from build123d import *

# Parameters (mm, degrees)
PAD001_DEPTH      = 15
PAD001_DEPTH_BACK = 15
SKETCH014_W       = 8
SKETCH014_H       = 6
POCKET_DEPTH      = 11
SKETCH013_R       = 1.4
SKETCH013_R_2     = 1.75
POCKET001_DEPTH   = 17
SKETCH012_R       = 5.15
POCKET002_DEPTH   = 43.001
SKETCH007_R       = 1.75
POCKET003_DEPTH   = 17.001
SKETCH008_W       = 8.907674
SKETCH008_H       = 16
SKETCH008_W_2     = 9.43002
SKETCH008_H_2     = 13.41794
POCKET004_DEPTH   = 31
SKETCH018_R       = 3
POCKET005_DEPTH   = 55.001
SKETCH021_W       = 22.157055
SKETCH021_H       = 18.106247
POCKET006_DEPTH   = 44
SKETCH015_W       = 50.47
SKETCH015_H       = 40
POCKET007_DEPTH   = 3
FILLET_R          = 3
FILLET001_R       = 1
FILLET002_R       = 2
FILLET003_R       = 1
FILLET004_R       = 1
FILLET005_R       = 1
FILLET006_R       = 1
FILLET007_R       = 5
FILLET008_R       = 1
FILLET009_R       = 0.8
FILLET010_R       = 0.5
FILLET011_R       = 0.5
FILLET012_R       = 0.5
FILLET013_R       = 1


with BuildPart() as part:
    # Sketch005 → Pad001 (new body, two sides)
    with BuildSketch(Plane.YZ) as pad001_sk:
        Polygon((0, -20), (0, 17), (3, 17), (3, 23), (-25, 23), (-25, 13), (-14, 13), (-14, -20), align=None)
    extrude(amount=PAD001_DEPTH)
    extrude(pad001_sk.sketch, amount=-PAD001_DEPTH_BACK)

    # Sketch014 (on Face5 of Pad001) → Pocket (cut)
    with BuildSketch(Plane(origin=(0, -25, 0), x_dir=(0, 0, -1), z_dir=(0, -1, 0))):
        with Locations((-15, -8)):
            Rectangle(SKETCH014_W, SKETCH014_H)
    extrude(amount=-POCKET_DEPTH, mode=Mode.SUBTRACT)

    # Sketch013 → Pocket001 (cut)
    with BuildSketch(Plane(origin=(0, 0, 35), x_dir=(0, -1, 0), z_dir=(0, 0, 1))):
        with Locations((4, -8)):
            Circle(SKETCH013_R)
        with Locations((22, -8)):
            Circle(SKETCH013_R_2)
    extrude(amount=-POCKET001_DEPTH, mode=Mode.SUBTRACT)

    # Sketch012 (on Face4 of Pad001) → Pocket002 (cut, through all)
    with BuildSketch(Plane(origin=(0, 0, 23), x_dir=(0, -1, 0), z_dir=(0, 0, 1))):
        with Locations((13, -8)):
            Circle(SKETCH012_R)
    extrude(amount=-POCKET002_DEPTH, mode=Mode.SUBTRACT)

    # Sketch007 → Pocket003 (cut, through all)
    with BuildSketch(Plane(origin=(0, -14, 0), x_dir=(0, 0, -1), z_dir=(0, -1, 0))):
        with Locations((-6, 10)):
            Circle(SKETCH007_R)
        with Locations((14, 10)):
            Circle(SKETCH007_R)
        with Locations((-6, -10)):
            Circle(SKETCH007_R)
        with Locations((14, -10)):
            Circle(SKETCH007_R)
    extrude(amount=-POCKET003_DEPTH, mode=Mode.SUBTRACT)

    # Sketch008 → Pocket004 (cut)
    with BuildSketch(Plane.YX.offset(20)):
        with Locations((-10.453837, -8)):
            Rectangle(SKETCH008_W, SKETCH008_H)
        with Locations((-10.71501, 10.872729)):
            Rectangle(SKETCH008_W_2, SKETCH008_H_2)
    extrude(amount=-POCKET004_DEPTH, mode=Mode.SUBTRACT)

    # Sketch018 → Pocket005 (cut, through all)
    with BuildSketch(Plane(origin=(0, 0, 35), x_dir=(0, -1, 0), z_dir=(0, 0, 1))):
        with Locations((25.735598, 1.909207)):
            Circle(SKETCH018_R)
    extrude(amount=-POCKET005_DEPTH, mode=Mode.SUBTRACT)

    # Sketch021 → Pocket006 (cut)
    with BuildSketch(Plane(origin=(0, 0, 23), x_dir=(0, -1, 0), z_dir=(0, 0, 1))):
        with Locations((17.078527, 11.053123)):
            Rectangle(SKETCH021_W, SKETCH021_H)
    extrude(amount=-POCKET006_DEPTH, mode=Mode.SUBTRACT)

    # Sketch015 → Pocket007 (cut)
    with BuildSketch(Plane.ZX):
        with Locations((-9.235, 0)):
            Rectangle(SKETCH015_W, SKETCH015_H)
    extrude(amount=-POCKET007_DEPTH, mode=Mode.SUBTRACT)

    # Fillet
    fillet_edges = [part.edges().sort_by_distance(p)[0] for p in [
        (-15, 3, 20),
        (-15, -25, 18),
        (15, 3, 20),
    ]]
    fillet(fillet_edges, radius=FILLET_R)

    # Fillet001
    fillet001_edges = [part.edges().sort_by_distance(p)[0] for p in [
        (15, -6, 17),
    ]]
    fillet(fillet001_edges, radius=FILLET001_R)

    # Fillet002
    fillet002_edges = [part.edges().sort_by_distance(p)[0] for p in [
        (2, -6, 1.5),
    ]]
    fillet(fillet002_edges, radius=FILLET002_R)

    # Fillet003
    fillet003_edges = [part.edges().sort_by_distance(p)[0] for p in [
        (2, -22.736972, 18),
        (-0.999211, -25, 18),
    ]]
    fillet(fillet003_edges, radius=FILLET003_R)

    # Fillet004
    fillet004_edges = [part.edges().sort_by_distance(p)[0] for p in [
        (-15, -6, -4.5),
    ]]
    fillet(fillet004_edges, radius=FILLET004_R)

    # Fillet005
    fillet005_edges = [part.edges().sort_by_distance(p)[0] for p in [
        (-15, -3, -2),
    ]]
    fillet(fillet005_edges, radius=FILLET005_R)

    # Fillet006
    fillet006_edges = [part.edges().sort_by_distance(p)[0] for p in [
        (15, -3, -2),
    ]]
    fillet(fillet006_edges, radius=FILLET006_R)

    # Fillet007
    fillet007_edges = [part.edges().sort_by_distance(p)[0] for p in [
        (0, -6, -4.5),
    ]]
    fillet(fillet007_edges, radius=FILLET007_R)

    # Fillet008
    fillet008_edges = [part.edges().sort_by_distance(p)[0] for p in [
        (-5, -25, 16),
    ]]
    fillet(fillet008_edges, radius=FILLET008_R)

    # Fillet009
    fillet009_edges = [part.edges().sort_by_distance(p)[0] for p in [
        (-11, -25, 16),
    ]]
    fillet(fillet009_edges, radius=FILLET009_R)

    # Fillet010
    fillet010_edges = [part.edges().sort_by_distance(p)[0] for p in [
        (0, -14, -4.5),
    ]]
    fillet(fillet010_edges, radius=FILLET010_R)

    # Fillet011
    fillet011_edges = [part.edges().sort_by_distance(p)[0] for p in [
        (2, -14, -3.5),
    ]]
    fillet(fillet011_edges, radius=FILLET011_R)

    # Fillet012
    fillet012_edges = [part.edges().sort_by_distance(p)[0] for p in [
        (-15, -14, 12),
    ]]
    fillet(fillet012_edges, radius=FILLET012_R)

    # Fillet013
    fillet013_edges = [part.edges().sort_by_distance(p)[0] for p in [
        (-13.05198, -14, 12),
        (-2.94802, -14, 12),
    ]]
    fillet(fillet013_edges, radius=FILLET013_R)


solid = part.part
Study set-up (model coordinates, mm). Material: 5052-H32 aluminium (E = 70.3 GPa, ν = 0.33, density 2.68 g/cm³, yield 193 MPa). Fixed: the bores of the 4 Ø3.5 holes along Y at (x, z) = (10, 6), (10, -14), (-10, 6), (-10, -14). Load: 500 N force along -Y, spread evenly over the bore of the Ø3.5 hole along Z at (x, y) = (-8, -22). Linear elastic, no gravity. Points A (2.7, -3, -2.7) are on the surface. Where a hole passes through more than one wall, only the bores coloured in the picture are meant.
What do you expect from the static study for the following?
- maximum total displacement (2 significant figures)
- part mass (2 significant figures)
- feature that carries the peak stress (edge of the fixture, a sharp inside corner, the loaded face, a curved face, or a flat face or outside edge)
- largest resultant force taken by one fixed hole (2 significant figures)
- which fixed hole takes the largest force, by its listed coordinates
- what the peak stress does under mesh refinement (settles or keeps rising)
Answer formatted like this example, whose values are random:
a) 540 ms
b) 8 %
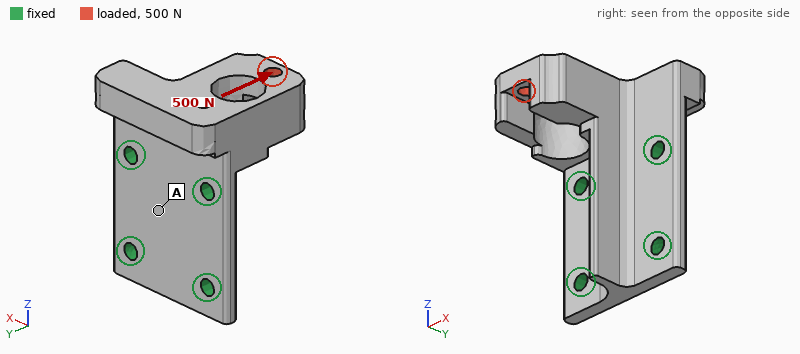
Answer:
a) 83 µm
b) 21 g
c) edge of the fixture
d) 580 N
e) (-10, 6)
f) keeps rising
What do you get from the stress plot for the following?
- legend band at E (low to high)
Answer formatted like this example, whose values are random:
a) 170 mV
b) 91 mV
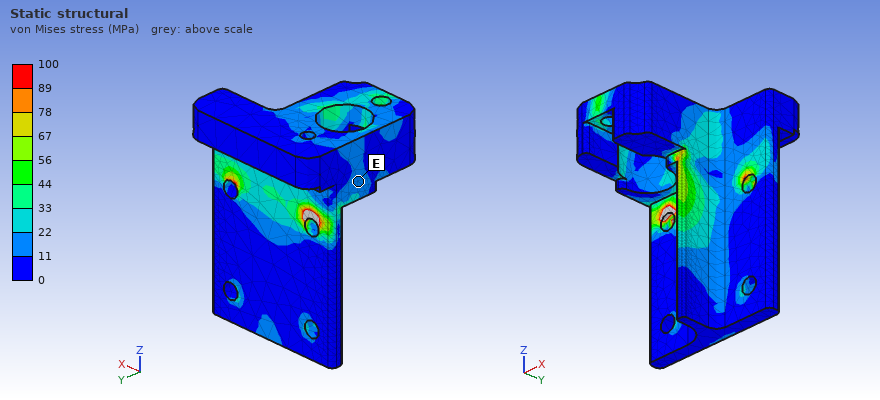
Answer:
a) 11 to 22 MPa
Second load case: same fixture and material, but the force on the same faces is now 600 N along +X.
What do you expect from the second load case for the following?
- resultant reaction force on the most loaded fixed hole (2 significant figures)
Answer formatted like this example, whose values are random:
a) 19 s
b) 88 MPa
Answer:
a) 720 N
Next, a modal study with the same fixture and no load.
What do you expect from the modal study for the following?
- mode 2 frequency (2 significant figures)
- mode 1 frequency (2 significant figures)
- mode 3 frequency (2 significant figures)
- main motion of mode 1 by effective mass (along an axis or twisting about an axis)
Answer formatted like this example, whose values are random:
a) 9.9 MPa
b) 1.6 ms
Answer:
a) 8200 Hz
b) 5200 Hz
c) 16 kHz
d) along Y
